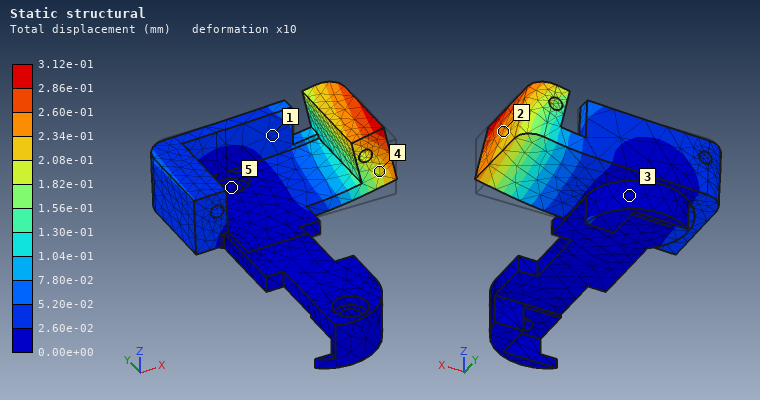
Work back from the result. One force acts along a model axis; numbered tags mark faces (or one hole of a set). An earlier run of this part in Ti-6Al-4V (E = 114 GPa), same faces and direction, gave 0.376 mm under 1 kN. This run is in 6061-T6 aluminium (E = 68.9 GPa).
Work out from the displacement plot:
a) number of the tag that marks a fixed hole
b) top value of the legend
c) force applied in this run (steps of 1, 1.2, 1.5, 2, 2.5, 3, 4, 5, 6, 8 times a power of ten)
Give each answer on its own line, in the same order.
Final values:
5
3.12e-01 mm
500 N
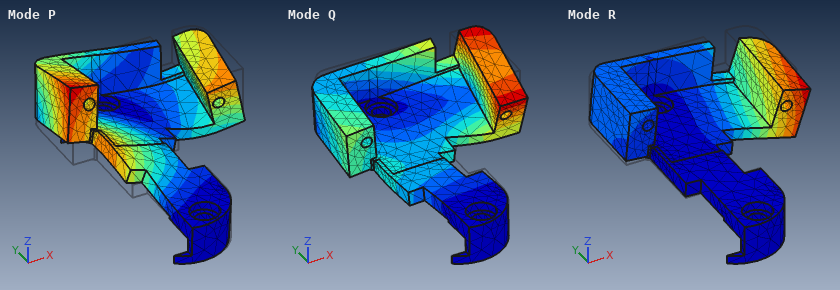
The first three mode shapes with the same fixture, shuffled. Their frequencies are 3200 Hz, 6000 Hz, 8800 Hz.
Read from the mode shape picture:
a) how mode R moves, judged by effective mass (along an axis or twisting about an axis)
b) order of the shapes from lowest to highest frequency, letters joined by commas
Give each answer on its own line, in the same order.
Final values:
along Z
R, Q, P
